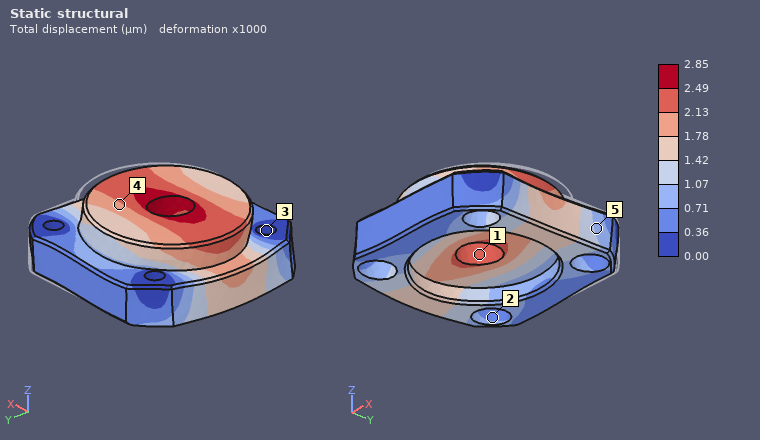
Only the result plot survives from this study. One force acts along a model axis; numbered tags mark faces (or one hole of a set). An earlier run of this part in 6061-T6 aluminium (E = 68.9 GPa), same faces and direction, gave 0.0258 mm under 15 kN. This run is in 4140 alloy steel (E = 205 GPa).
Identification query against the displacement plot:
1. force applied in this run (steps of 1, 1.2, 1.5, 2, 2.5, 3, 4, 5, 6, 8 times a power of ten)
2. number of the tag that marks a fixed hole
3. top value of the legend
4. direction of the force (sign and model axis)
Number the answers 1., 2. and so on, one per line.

1. 5 kN
2. 3
3. 2.85 µm
4. -X
